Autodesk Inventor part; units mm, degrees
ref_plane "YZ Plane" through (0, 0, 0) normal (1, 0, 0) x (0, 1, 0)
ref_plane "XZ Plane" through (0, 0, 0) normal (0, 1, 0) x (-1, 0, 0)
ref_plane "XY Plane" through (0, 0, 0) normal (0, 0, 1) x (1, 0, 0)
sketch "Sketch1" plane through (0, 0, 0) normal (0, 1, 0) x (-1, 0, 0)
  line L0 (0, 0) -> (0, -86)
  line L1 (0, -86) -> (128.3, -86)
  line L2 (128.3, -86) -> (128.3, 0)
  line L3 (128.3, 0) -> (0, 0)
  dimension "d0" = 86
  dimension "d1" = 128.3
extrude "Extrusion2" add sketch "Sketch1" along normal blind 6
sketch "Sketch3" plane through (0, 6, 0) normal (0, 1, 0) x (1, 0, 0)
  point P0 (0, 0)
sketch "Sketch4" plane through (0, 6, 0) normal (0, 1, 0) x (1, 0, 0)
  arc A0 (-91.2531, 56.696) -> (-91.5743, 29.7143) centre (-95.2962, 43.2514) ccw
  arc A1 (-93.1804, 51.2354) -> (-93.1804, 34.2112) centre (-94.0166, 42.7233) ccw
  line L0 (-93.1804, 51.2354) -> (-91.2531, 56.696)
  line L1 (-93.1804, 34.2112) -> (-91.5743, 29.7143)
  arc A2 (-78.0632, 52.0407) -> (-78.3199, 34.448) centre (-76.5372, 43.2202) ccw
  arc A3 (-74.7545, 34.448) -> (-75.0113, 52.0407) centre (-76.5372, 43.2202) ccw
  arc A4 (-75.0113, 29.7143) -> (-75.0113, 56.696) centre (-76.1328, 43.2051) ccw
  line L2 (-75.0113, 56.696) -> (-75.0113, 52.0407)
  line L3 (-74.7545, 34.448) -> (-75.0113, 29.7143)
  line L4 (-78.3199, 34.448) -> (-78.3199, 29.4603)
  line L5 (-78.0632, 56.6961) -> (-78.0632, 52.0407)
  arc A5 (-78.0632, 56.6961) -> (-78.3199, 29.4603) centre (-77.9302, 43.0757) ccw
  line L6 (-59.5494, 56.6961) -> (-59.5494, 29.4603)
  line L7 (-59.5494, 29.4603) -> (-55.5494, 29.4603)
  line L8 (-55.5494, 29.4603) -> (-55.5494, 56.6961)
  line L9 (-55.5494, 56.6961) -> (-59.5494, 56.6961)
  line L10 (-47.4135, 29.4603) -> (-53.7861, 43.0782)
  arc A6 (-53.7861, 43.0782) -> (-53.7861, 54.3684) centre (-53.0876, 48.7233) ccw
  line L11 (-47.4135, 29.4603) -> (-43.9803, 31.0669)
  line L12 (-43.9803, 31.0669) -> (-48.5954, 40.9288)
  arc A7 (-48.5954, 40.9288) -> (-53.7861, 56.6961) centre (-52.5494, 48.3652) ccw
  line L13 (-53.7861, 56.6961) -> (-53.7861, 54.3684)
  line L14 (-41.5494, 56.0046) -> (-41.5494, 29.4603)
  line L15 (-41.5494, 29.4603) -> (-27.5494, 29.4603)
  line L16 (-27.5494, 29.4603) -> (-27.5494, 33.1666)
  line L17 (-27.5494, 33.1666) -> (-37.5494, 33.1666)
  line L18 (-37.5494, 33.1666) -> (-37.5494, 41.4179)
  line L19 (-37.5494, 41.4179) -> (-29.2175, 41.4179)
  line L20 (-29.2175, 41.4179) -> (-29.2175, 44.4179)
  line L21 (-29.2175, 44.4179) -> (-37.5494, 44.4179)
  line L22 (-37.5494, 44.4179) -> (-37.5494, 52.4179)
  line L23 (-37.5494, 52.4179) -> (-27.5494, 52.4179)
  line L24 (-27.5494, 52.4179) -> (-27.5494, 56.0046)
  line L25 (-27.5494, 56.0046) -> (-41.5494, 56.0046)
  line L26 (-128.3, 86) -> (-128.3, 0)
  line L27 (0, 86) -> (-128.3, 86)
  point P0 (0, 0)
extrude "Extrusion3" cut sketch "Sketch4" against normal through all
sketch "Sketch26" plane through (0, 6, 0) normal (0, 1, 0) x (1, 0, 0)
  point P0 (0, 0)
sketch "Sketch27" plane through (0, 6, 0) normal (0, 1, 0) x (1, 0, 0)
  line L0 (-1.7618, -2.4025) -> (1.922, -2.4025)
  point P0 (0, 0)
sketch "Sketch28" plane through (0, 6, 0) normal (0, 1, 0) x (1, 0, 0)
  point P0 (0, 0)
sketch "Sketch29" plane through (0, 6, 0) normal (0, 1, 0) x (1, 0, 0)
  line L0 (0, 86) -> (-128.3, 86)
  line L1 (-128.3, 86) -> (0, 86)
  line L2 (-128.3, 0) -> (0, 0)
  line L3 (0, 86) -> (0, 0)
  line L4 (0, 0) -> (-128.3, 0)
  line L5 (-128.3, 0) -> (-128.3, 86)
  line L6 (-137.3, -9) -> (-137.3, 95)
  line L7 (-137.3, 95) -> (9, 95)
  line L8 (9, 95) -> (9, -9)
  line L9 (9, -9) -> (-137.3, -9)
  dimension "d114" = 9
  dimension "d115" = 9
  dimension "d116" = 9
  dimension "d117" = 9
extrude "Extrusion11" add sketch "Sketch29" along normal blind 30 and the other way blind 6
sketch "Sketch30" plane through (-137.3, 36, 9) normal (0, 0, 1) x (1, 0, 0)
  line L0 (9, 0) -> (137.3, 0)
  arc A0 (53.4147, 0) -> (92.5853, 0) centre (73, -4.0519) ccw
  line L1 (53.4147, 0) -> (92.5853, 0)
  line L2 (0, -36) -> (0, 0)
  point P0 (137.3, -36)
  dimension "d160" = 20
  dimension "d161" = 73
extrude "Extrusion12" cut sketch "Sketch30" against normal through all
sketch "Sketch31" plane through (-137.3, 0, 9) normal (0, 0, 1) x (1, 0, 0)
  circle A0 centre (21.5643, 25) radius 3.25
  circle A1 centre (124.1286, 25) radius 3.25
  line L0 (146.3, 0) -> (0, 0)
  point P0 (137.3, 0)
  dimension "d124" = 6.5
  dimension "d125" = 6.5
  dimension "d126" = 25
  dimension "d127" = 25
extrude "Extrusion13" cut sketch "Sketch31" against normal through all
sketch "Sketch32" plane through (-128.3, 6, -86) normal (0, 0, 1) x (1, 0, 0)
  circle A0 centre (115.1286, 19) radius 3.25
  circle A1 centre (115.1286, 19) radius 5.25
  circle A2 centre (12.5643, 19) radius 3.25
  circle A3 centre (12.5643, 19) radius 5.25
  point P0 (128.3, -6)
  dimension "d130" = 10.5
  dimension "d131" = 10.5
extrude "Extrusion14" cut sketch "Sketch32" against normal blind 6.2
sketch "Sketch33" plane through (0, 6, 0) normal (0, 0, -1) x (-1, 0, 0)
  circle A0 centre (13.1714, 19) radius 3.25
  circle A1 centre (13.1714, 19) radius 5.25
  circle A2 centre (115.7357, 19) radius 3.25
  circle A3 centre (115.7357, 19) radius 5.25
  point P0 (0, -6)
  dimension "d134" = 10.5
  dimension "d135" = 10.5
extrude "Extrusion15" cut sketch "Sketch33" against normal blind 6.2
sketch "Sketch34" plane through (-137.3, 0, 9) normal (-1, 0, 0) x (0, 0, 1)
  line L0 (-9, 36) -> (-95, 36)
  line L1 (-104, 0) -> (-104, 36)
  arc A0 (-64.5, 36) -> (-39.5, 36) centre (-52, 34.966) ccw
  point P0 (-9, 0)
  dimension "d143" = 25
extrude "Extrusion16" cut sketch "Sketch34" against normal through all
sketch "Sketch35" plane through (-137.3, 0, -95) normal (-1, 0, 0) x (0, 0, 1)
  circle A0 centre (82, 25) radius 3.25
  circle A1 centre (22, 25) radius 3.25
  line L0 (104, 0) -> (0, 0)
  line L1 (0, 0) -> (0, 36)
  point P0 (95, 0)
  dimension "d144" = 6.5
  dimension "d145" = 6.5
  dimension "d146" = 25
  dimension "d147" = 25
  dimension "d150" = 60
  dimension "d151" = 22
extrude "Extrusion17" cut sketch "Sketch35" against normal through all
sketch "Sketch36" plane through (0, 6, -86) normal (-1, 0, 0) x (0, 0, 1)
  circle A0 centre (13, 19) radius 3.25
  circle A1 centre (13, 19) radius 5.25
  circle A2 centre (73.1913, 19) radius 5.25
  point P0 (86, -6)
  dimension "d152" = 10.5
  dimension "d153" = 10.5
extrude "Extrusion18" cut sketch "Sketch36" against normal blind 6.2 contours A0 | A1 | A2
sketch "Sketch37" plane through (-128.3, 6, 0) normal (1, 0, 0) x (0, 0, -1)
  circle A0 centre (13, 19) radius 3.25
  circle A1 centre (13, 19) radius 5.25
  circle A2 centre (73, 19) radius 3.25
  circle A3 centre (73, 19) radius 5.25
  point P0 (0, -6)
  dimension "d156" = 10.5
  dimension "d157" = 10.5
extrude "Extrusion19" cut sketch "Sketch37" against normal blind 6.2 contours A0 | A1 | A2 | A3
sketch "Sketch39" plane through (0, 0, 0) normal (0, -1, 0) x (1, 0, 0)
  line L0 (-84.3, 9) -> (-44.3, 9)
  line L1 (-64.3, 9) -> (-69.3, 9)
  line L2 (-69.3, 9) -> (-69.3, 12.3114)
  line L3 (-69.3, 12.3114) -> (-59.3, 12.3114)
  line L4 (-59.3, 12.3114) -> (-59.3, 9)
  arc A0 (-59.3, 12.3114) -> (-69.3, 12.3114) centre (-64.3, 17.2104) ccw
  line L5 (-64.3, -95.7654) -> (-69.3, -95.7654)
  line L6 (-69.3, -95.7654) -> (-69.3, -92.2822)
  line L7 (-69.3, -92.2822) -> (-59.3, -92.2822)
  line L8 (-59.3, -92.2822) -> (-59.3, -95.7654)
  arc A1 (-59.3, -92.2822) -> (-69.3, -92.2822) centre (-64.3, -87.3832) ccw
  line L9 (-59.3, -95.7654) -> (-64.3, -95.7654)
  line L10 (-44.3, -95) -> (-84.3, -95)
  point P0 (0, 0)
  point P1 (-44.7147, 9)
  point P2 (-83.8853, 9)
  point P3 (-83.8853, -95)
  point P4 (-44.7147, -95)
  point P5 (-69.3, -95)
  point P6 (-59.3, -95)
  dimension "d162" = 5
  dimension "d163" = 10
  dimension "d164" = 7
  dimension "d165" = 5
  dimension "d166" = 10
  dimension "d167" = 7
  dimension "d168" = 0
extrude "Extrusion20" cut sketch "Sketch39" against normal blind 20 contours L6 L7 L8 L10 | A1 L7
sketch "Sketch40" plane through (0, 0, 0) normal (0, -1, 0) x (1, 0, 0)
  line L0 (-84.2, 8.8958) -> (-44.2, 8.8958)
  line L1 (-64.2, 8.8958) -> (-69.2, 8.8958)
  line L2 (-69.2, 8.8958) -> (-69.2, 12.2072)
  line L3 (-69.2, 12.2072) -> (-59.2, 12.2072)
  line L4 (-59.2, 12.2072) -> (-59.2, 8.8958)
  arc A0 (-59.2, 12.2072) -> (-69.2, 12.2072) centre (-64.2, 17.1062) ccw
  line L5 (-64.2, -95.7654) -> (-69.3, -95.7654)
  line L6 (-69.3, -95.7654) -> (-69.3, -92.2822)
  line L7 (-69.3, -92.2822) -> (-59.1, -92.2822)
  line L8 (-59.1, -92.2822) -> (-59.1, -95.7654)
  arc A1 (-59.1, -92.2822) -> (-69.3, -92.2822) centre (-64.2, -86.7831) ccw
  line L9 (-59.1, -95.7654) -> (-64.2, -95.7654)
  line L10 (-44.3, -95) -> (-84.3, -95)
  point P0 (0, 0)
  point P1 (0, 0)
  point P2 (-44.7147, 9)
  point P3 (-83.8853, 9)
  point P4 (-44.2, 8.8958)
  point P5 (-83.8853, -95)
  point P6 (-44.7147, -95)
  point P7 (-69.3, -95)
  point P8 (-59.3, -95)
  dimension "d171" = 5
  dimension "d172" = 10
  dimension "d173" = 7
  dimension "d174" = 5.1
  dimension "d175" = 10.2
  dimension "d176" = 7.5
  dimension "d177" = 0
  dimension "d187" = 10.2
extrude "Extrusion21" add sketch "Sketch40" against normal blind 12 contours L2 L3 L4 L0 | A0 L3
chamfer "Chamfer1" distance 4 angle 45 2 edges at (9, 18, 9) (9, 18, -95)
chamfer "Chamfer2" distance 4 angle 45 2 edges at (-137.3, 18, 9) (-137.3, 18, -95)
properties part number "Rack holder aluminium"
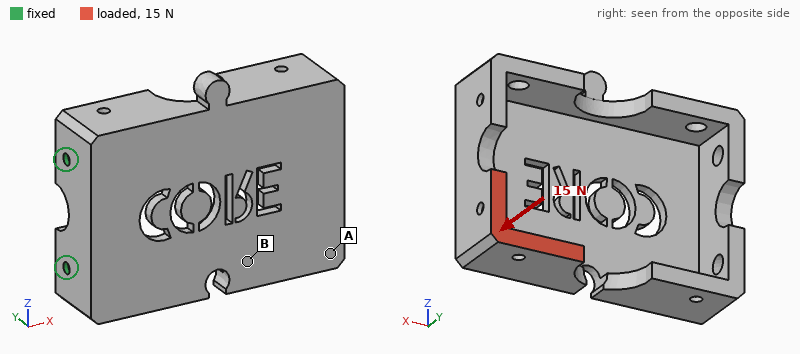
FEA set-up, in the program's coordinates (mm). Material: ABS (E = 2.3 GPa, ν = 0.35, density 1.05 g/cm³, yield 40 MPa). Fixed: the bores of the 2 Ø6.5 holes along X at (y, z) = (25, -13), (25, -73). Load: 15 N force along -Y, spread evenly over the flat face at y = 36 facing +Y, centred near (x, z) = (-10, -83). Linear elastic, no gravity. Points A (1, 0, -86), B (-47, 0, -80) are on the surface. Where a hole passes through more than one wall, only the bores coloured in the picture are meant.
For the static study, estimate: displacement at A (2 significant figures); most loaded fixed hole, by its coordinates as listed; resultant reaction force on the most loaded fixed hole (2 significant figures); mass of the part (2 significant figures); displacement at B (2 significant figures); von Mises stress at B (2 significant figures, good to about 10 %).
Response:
1.7 mm
(25, -73)
19 N
190 g
0.97 mm
0.81 MPa
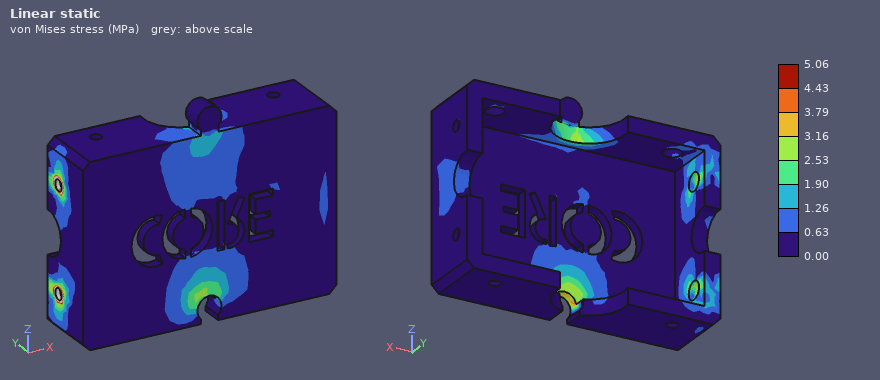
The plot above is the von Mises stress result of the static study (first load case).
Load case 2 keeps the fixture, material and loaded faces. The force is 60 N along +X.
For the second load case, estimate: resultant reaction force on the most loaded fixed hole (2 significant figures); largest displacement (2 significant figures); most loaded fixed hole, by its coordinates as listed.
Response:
67 N
2.0 mm
(25, -73)
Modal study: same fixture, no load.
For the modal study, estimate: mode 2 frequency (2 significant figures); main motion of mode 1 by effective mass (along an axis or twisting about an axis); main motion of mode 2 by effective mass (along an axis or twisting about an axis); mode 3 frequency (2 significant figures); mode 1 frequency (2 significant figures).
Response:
120 Hz
along Y
along Z
260 Hz
56 Hz
